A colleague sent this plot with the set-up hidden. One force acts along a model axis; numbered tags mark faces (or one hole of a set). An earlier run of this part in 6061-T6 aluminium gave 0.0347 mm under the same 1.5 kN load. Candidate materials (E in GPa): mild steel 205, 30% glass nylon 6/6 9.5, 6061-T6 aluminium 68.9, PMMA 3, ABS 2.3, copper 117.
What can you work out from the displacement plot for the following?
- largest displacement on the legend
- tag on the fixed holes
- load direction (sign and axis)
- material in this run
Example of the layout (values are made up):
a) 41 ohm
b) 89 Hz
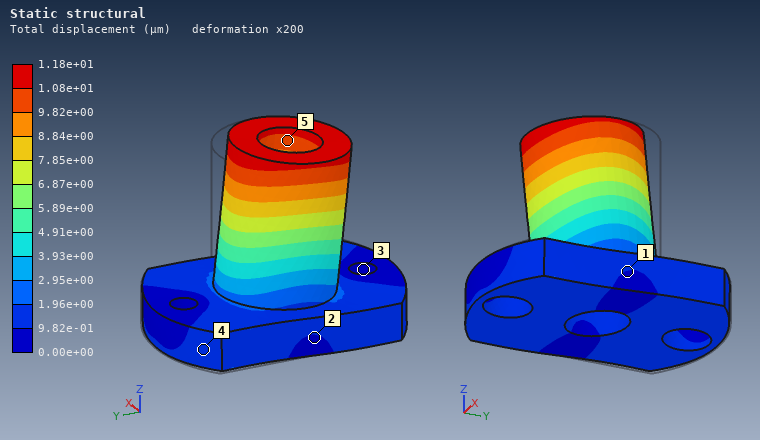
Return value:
a) 1.18e+01 µm
b) 3
c) -Y
d) mild steel
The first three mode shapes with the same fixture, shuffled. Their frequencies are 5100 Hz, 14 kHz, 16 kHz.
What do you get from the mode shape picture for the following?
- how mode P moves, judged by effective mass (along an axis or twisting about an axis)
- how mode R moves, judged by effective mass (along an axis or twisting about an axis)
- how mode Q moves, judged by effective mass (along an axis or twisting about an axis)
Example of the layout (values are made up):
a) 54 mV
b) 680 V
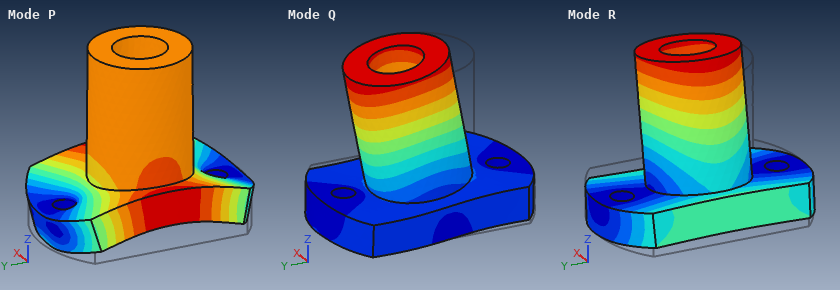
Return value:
a) along Z
b) along X
c) along Y
